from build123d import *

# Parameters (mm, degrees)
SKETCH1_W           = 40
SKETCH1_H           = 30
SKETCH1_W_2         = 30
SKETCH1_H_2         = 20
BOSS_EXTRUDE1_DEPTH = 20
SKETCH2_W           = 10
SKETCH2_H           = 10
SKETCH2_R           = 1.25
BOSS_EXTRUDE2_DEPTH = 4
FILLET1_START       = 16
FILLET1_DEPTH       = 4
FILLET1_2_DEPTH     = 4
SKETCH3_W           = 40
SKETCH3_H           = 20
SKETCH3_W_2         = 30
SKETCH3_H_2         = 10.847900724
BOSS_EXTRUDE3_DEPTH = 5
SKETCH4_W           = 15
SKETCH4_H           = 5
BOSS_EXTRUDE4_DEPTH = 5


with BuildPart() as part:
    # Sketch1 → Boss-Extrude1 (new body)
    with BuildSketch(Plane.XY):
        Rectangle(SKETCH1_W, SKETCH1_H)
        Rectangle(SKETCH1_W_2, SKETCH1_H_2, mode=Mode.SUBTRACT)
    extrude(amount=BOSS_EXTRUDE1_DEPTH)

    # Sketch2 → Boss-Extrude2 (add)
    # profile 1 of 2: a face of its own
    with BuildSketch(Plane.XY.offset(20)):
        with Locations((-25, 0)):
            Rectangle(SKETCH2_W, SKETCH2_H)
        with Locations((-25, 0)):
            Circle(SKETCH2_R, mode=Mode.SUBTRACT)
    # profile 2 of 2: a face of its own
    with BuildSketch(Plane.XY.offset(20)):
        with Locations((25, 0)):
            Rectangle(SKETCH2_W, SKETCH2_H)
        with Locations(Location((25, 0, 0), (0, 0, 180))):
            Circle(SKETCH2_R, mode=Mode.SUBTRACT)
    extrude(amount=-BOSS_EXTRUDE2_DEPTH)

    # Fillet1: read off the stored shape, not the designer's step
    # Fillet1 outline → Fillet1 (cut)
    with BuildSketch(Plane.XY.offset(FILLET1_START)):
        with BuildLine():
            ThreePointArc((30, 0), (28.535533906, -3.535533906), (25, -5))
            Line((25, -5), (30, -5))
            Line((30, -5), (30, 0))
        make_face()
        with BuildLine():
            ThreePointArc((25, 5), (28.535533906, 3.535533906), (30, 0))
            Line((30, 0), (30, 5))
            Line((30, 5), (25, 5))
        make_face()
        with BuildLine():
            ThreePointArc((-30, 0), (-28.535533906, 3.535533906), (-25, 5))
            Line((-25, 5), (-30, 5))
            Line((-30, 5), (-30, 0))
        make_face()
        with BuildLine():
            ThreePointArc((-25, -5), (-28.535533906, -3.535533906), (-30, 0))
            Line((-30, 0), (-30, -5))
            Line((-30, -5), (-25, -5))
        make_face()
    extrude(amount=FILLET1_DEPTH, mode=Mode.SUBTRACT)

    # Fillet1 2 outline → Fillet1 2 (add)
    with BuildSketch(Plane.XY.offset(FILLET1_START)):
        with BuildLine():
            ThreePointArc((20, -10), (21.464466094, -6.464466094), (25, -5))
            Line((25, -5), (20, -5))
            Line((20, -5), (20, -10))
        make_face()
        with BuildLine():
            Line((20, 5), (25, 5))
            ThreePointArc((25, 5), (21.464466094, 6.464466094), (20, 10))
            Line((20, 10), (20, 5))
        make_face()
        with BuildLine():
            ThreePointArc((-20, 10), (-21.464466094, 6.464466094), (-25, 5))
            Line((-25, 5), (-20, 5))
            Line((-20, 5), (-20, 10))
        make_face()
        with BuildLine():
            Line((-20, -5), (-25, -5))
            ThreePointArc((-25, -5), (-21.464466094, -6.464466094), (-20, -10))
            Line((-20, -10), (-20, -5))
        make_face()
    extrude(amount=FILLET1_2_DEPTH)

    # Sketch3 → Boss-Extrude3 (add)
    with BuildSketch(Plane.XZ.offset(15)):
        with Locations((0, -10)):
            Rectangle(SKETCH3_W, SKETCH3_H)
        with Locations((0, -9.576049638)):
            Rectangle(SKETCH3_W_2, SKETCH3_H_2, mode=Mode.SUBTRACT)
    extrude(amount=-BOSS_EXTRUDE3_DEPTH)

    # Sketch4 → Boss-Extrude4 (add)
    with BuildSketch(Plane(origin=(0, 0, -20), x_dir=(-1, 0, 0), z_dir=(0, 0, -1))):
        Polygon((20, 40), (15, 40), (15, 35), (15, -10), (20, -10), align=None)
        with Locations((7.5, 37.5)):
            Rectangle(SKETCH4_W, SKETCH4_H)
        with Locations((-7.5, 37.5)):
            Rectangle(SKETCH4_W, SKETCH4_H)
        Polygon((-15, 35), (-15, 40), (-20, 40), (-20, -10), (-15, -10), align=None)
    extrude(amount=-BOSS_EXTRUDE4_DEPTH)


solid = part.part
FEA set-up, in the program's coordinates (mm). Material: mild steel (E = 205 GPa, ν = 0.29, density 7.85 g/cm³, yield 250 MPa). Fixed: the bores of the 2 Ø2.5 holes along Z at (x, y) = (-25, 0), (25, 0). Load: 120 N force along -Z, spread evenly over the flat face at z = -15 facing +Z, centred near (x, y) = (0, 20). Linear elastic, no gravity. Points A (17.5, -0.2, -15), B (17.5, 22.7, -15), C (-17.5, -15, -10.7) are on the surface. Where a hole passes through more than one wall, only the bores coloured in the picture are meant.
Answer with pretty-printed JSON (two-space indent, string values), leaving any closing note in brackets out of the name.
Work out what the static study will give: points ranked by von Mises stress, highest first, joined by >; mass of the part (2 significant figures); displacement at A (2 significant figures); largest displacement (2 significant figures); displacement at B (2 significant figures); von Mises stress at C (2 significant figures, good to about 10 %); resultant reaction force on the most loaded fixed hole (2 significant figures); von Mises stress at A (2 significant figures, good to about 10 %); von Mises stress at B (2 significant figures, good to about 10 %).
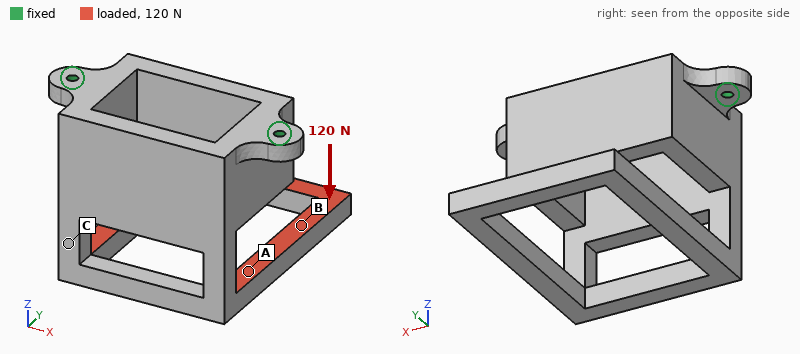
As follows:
{
  "points ranked by von Mises stress, highest first, joined by >": "C > A > B",
  "mass of the part": "140 g",
  "displacement at A": "0.060 mm",
  "largest displacement": "0.32 mm",
  "displacement at B": "0.20 mm",
  "von Mises stress at C": "94 MPa",
  "resultant reaction force on the most loaded fixed hole": "60 N",
  "von Mises stress at A": "61 MPa",
  "von Mises stress at B": "16 MPa"
}
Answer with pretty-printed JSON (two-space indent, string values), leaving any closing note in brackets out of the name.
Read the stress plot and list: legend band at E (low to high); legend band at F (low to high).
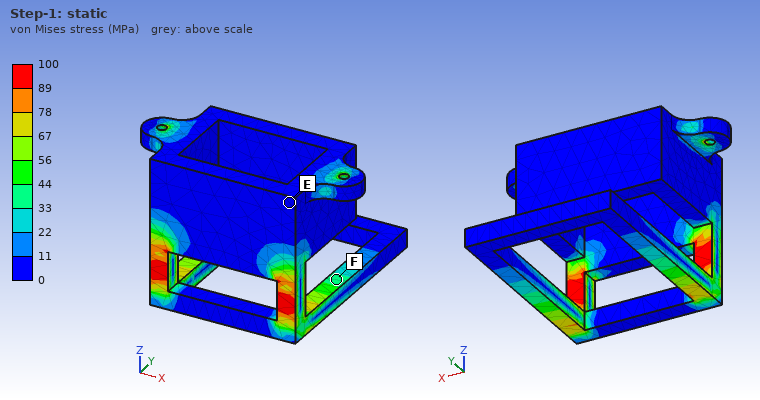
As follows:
{
  "legend band at E": "0 to 11 MPa",
  "legend band at F": "33 to 44 MPa"
}
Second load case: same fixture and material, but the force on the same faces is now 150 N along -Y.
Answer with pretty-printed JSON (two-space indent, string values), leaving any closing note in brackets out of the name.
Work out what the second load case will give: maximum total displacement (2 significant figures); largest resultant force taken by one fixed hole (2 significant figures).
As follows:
{
  "maximum total displacement": "82 µm",
  "largest resultant force taken by one fixed hole": "76 N"
}
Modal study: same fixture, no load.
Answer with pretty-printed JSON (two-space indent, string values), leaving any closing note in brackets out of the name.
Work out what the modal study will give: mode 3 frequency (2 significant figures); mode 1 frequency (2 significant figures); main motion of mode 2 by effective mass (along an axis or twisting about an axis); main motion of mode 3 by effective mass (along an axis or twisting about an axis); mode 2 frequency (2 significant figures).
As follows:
{
  "mode 3 frequency": "1500 Hz",
  "mode 1 frequency": "670 Hz",
  "main motion of mode 2 by effective mass": "along X",
  "main motion of mode 3 by effective mass": "along Y",
  "mode 2 frequency": "1200 Hz"
}
